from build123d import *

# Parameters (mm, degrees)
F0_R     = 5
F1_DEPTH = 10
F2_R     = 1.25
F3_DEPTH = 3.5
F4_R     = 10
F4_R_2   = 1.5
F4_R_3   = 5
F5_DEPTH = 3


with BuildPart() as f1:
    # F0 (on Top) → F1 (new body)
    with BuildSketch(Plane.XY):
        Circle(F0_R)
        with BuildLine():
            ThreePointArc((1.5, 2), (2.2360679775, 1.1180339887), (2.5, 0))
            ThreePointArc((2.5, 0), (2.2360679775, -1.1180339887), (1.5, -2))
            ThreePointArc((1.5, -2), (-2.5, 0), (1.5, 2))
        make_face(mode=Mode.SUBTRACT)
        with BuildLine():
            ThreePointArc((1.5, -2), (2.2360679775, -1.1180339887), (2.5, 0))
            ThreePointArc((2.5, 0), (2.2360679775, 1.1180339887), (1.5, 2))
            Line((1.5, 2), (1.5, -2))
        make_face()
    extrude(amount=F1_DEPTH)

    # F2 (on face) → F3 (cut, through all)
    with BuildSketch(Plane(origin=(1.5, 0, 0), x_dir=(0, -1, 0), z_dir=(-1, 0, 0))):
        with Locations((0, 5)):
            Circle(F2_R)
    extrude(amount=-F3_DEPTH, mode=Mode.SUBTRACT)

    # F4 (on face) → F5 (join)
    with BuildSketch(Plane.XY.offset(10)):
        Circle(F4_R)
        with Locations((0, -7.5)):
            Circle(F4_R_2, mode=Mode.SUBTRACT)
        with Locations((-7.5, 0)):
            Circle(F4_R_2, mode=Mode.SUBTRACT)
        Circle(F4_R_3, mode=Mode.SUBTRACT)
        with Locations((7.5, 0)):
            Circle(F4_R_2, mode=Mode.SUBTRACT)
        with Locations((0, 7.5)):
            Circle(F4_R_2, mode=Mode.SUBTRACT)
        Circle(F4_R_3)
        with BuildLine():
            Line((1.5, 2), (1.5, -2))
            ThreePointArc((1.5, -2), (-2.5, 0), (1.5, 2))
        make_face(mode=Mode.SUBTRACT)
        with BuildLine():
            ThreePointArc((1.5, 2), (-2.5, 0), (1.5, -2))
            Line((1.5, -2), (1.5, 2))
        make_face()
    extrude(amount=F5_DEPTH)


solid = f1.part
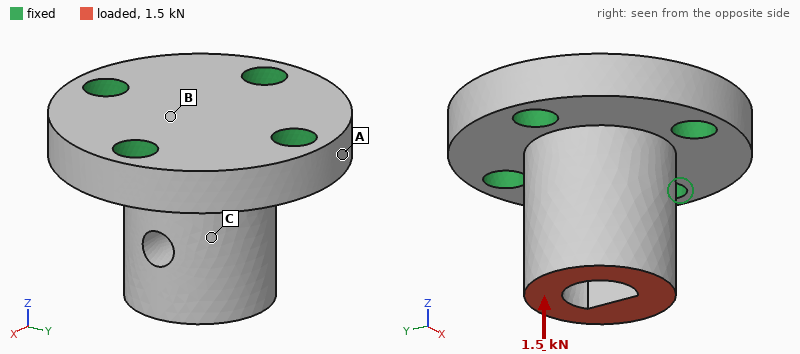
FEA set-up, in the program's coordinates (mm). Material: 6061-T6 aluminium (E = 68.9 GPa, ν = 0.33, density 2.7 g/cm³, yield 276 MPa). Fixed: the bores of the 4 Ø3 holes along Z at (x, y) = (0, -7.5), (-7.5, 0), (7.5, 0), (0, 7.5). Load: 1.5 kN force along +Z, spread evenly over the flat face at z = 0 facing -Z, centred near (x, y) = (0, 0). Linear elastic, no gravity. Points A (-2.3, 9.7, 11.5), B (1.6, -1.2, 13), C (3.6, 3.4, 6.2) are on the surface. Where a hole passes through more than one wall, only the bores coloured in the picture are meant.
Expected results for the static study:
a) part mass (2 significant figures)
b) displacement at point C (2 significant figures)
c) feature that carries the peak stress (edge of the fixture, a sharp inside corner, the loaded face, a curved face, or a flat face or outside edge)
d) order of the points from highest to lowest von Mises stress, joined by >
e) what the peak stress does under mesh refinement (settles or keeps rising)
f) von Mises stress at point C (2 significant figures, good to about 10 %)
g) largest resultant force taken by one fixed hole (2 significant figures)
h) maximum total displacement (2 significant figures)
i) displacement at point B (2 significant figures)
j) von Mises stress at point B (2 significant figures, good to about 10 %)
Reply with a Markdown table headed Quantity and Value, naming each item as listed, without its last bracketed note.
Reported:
| Quantity | Value |
|---|---|
| part mass | 3.9 g |
| displacement at point C | 4.6 µm |
| feature that carries the peak stress | edge of the fixture |
| order of the points from highest to lowest von Mises stress, joined by > | C > B > A |
| what the peak stress does under mesh refinement | keeps rising |
| von Mises stress at point C | 28 MPa |
| largest resultant force taken by one fixed hole | 400 N |
| maximum total displacement | 7.8 µm |
| displacement at point B | 3.2 µm |
| von Mises stress at point B | 18 MPa |
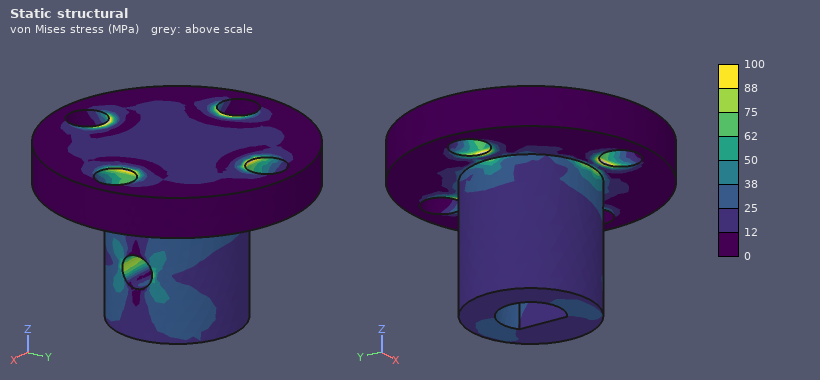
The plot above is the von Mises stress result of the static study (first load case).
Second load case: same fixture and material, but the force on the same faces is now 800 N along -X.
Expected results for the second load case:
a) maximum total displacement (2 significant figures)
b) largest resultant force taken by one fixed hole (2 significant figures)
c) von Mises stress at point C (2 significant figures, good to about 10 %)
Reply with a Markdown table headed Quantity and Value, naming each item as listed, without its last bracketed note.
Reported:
| Quantity | Value |
|---|---|
| maximum total displacement | 33 µm |
| largest resultant force taken by one fixed hole | 750 N |
| von Mises stress at point C | 47 MPa |
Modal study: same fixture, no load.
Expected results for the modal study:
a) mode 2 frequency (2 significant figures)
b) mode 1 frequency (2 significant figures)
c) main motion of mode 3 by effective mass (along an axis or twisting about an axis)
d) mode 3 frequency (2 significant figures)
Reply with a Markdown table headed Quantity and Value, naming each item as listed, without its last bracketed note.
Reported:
| Quantity | Value |
|---|---|
| mode 2 frequency | 35 kHz |
| mode 1 frequency | 35 kHz |
| main motion of mode 3 by effective mass | along Z |
| mode 3 frequency | 67 kHz |
